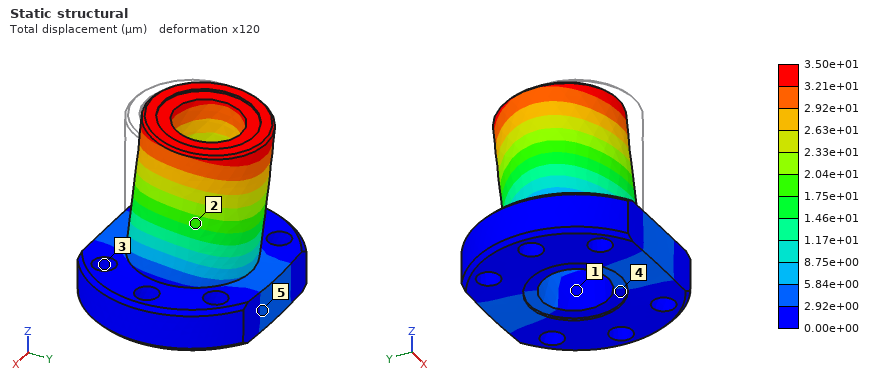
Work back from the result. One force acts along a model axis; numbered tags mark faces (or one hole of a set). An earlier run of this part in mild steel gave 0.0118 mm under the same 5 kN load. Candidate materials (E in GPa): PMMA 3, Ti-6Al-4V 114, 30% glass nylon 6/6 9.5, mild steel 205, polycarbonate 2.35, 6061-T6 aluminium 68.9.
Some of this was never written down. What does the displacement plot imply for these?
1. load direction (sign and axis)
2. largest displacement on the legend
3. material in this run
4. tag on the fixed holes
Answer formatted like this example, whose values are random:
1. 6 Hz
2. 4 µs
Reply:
1. +Y
2. 3.50e+01 µm
3. 6061-T6 aluminium
4. 3
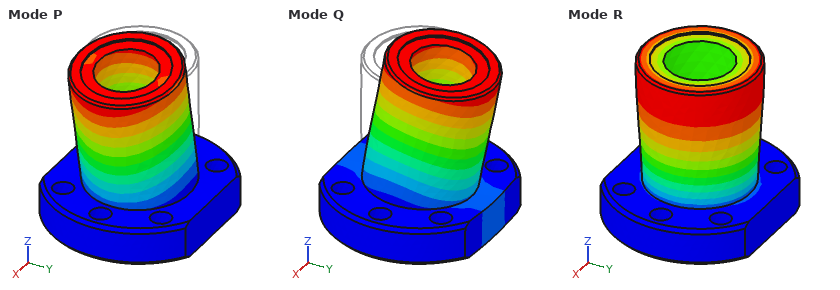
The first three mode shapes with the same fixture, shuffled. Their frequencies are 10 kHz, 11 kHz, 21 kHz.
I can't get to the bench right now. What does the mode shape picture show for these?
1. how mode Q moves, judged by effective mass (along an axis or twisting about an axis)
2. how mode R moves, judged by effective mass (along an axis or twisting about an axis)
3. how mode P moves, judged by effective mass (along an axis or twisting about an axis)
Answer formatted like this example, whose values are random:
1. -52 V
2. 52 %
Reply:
1. along Y
2. twisting about Z
3. along X
